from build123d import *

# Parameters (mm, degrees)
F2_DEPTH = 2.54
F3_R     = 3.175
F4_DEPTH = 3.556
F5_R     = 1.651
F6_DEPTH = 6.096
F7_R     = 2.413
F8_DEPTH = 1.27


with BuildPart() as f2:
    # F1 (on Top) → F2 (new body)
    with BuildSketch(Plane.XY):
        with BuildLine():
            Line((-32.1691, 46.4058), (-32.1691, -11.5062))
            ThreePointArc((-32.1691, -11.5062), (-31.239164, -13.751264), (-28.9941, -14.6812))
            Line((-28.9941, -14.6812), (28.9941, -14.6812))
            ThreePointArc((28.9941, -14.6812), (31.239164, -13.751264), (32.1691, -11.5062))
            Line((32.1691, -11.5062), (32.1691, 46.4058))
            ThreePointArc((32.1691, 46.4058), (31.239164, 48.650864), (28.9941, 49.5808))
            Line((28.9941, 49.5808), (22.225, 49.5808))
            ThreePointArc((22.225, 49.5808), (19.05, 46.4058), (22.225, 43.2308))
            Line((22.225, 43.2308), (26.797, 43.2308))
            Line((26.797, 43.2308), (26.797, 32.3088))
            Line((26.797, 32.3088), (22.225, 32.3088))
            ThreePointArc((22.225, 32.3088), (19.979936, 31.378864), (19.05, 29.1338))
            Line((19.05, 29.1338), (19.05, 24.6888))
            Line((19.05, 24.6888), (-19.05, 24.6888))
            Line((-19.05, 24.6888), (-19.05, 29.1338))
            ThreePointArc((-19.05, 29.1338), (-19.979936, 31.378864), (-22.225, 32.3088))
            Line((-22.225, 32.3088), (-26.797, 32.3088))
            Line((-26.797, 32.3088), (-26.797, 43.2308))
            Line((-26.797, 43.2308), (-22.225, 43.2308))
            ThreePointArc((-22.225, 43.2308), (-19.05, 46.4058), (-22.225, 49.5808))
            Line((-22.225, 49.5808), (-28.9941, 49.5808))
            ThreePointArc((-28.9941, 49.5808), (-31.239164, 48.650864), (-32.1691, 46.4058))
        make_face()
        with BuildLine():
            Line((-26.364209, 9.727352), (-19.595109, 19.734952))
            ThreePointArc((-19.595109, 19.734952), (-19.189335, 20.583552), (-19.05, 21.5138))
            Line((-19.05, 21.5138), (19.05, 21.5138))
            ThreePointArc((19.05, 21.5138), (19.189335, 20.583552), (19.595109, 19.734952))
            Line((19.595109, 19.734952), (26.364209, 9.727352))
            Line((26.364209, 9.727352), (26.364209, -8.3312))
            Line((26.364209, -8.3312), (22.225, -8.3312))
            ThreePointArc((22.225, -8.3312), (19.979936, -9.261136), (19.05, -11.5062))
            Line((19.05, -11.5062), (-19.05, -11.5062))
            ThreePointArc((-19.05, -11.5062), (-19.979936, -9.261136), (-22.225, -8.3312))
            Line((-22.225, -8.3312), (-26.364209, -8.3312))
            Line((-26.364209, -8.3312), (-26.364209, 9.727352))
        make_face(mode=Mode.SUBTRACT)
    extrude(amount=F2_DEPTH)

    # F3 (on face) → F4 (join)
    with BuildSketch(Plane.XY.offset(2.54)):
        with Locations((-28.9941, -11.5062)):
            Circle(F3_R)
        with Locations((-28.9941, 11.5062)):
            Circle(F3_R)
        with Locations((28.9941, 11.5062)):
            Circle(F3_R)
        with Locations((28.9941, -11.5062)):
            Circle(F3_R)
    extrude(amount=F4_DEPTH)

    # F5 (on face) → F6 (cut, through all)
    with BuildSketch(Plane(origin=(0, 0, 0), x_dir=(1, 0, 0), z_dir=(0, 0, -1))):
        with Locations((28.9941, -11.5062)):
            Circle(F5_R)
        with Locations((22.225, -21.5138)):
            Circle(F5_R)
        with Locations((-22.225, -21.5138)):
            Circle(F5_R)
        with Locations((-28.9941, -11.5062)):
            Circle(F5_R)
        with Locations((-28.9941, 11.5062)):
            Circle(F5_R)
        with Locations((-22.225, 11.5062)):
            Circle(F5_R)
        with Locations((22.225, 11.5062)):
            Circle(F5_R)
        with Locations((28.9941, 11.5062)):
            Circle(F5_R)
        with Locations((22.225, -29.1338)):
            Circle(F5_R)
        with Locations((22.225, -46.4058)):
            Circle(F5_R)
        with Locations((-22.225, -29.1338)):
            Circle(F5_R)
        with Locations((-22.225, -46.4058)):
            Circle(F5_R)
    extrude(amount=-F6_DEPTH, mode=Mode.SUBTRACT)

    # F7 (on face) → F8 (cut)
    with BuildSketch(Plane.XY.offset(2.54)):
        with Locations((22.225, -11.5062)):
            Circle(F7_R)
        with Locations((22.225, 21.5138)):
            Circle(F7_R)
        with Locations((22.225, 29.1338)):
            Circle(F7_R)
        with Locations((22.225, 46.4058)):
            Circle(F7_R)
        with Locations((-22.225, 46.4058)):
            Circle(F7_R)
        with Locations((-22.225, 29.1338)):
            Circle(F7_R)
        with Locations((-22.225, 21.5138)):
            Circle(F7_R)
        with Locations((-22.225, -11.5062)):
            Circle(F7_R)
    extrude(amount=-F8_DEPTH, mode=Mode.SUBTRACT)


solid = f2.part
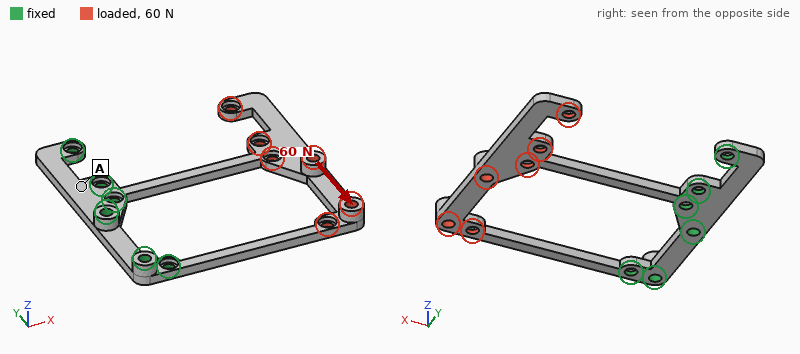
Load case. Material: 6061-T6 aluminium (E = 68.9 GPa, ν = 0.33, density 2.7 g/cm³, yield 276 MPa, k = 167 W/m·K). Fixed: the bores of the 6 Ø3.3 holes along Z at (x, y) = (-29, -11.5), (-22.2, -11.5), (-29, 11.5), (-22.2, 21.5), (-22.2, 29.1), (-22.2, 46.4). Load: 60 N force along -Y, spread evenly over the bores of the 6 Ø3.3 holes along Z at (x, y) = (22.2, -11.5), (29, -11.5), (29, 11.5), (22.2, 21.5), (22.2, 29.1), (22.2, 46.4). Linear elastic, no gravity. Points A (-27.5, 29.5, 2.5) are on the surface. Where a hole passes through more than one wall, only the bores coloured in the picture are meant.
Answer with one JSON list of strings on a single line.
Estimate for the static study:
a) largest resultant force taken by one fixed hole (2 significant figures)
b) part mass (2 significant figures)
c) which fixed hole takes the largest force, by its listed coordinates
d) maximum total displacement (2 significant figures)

["98 N", "9.4 g", "(-22.2, 29.1)", "0.49 mm"]
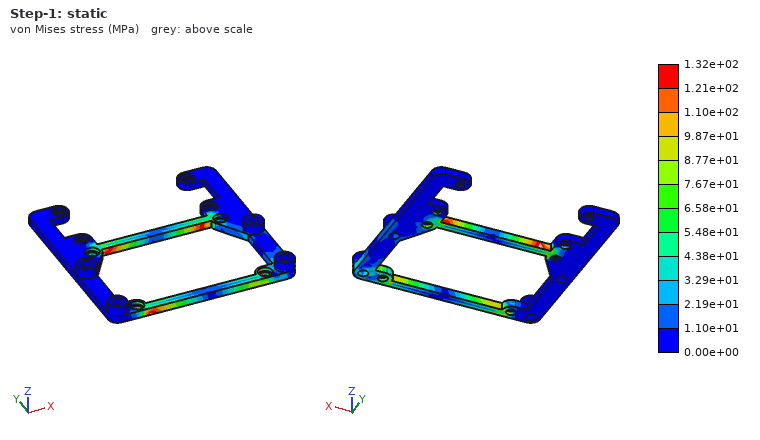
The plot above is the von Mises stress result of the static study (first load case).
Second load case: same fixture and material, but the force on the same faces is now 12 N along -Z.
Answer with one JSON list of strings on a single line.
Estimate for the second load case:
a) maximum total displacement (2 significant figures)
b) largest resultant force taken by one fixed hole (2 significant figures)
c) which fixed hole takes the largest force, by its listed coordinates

["0.95 mm", "37 N", "(-22.2, 21.5)"]
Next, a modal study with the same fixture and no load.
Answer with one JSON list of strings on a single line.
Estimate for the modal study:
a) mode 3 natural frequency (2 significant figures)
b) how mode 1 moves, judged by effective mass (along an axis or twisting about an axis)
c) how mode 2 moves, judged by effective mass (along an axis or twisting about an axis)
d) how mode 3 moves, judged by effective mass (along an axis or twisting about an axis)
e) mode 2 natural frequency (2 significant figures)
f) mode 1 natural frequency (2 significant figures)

["870 Hz", "along Z", "twisting about X", "along Y", "640 Hz", "280 Hz"]
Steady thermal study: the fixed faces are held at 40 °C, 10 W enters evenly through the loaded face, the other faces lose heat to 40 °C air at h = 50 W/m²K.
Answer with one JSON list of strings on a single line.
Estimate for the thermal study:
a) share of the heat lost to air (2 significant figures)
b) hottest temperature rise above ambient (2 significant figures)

["66 %", "74 K"]
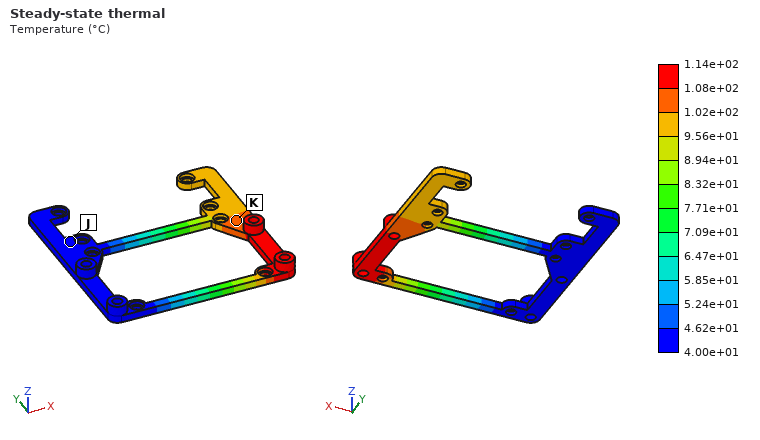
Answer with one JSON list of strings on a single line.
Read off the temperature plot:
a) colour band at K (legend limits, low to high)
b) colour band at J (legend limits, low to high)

["1.02e+02 to 1.08e+02 °C", "4.00e+01 to 4.62e+01 °C"]
